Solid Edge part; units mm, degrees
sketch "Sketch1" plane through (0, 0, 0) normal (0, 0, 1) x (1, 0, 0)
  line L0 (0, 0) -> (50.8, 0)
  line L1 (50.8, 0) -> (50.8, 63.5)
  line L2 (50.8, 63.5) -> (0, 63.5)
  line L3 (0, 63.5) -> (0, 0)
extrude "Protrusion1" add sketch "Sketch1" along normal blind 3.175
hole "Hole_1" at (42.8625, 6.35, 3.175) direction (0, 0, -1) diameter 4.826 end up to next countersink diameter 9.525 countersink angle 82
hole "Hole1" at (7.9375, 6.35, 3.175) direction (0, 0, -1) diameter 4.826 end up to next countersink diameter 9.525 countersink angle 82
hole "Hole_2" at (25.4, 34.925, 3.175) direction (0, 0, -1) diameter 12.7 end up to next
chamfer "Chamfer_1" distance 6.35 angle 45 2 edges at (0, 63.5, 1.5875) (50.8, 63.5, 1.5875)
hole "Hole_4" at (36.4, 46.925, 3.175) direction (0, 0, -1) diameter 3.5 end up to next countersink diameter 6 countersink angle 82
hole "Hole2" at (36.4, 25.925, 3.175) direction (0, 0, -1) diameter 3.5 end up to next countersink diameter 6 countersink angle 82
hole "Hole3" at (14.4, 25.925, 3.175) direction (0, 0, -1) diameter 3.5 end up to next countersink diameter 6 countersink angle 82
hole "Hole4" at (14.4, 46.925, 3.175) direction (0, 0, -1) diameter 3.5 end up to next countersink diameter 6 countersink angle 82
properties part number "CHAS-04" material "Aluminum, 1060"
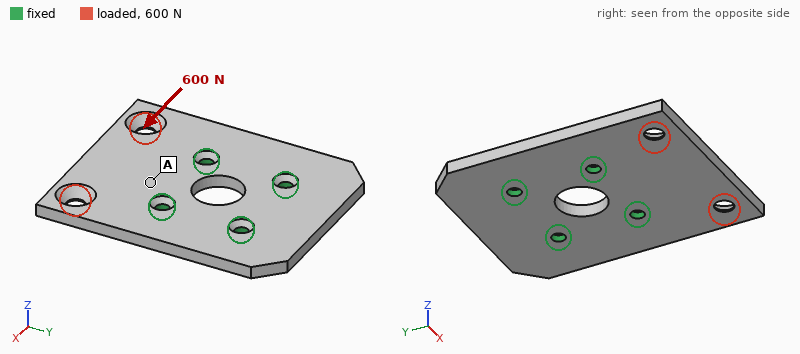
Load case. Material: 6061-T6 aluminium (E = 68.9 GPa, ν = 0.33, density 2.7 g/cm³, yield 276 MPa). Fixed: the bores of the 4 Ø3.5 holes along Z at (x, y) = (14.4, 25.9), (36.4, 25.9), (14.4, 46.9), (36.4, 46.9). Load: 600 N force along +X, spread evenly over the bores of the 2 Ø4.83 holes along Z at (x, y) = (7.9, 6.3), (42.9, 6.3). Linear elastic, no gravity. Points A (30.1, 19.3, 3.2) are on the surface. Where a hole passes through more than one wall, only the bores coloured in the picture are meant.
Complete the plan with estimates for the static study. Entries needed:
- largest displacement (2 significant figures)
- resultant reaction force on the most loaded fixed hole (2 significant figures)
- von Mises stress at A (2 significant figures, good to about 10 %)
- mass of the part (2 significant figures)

27 µm
440 N
7.0 MPa
25 g
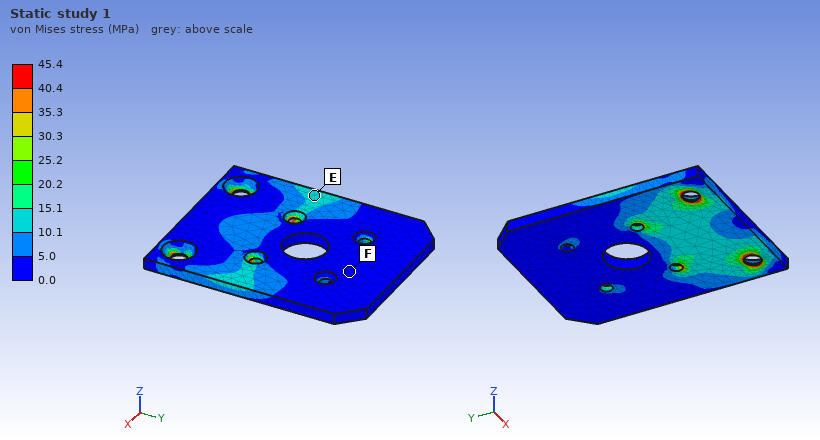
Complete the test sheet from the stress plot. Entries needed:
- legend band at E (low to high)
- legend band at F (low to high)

10.1 to 15.1 MPa
0.0 to 5.0 MPa
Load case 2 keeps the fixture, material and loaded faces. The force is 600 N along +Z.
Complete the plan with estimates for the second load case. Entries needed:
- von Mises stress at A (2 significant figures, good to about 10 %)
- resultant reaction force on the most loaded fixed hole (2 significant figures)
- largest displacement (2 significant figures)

83 MPa
540 N
0.35 mm
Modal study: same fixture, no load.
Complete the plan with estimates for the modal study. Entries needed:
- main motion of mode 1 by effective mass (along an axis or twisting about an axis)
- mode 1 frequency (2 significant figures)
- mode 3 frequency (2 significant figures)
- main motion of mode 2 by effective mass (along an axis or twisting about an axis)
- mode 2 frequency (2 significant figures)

along Z
3400 Hz
7600 Hz
twisting about Y
5000 Hz
